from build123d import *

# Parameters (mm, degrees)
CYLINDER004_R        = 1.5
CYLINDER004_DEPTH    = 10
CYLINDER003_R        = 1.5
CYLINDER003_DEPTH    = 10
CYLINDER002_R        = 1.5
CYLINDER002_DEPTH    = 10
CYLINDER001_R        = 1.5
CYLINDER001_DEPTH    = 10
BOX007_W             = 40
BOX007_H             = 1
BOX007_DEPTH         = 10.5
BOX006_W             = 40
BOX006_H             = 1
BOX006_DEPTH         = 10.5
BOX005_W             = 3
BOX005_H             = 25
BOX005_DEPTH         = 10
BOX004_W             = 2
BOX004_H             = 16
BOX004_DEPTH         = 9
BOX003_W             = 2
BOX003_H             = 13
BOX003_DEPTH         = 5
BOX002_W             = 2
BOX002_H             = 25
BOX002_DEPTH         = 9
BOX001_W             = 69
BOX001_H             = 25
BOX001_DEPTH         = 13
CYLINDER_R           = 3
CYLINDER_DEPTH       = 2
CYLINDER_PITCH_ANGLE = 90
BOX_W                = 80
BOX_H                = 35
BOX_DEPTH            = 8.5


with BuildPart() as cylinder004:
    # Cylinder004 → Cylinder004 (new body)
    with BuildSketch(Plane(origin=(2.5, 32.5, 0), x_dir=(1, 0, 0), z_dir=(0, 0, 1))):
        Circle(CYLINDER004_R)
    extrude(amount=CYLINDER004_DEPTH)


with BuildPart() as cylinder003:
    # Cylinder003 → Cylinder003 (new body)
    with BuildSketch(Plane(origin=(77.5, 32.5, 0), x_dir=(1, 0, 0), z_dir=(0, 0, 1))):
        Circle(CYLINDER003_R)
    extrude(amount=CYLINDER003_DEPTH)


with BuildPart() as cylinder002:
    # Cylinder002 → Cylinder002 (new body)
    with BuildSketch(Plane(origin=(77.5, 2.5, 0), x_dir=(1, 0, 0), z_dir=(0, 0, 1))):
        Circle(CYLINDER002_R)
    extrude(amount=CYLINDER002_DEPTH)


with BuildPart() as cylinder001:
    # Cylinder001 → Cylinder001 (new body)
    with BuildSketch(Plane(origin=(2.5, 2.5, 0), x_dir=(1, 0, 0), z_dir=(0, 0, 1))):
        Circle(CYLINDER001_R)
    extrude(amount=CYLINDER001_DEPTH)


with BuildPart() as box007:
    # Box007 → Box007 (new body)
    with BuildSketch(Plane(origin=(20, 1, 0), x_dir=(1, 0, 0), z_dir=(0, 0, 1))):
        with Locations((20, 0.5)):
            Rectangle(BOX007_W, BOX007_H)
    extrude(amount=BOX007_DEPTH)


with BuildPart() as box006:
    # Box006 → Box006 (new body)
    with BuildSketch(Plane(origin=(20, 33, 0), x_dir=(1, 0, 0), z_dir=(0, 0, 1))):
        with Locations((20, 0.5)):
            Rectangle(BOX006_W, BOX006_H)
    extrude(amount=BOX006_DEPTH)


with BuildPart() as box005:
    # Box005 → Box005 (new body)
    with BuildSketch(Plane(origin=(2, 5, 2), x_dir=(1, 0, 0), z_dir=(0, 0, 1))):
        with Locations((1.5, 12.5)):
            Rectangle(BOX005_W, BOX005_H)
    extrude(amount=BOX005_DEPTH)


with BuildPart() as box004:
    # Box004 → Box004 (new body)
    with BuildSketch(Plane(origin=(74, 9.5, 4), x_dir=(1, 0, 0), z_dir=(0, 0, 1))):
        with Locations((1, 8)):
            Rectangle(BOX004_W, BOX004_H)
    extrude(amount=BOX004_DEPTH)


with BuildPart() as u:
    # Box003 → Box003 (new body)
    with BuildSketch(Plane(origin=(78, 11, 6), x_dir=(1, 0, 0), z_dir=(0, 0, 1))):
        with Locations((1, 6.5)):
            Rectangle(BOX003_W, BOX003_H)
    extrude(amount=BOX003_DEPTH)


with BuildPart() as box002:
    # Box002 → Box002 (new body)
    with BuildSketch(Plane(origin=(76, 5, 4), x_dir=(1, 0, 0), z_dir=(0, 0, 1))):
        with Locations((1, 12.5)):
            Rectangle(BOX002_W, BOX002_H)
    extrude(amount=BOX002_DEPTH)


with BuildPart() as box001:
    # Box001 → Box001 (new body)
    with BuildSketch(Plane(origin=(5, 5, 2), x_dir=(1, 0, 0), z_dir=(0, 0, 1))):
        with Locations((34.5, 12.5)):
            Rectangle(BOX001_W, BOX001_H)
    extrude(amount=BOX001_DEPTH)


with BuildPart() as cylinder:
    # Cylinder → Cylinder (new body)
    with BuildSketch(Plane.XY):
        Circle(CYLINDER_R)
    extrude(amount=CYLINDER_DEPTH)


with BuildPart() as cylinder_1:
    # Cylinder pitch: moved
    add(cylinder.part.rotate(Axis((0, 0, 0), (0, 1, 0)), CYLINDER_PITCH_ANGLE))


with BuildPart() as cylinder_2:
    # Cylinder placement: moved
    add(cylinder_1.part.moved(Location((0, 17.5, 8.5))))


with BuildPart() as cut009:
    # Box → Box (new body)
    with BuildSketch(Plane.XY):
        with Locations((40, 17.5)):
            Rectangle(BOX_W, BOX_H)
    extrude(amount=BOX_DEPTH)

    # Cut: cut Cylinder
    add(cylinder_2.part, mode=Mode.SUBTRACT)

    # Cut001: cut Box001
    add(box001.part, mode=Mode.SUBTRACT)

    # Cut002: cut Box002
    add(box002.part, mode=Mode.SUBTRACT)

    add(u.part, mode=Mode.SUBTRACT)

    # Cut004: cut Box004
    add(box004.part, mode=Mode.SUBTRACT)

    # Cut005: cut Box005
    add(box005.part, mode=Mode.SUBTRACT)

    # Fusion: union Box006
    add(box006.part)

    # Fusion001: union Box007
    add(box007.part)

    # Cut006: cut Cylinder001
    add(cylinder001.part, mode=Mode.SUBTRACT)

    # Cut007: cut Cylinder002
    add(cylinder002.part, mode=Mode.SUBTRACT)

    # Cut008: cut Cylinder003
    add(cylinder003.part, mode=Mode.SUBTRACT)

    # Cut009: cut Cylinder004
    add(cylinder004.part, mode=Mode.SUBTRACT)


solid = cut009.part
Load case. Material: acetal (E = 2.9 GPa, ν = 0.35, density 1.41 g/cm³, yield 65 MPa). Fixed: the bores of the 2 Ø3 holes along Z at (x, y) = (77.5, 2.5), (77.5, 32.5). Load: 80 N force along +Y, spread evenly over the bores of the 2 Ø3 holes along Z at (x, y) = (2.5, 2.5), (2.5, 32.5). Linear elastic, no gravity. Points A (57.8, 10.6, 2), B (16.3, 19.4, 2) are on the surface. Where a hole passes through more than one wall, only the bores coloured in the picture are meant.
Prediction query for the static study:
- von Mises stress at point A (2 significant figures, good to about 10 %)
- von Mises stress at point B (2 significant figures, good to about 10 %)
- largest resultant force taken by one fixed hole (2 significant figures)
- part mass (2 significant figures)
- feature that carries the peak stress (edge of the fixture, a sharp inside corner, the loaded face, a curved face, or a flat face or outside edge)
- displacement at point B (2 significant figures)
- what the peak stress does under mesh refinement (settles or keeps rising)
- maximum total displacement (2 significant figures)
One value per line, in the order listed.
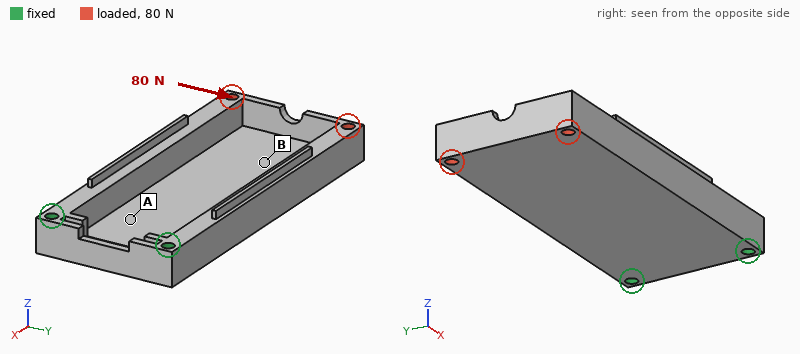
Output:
4.3 MPa
5.5 MPa
200 N
16 g
edge of the fixture
0.30 mm
keeps rising
0.96 mm
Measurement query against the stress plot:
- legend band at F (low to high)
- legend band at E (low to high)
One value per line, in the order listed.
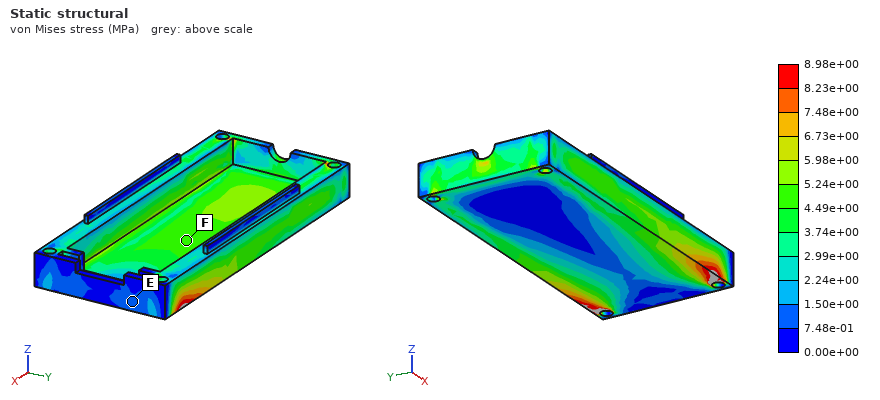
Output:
4.49e+00 to 5.24e+00 MPa
7.48e-01 to 1.50e+00 MPa
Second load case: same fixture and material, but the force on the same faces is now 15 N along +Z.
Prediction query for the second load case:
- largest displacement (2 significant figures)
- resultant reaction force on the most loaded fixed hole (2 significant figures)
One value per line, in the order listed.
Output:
0.92 mm
20 N
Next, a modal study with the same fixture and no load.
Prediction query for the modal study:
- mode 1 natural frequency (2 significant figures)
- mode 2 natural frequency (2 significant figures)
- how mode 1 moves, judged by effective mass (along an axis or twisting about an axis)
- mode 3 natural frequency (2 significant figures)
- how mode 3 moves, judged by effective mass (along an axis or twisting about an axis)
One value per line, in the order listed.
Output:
310 Hz
580 Hz
along Z
1300 Hz
along Y
